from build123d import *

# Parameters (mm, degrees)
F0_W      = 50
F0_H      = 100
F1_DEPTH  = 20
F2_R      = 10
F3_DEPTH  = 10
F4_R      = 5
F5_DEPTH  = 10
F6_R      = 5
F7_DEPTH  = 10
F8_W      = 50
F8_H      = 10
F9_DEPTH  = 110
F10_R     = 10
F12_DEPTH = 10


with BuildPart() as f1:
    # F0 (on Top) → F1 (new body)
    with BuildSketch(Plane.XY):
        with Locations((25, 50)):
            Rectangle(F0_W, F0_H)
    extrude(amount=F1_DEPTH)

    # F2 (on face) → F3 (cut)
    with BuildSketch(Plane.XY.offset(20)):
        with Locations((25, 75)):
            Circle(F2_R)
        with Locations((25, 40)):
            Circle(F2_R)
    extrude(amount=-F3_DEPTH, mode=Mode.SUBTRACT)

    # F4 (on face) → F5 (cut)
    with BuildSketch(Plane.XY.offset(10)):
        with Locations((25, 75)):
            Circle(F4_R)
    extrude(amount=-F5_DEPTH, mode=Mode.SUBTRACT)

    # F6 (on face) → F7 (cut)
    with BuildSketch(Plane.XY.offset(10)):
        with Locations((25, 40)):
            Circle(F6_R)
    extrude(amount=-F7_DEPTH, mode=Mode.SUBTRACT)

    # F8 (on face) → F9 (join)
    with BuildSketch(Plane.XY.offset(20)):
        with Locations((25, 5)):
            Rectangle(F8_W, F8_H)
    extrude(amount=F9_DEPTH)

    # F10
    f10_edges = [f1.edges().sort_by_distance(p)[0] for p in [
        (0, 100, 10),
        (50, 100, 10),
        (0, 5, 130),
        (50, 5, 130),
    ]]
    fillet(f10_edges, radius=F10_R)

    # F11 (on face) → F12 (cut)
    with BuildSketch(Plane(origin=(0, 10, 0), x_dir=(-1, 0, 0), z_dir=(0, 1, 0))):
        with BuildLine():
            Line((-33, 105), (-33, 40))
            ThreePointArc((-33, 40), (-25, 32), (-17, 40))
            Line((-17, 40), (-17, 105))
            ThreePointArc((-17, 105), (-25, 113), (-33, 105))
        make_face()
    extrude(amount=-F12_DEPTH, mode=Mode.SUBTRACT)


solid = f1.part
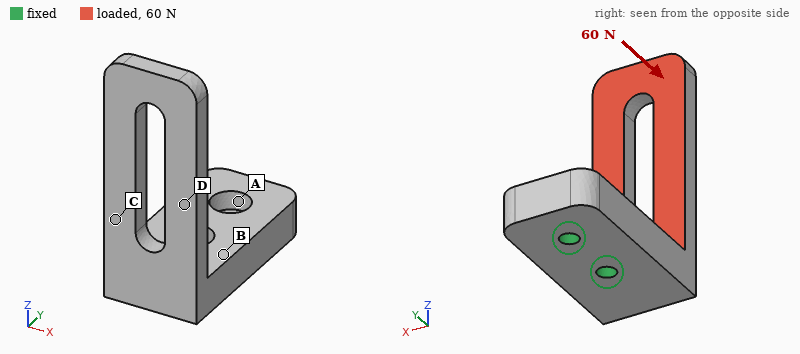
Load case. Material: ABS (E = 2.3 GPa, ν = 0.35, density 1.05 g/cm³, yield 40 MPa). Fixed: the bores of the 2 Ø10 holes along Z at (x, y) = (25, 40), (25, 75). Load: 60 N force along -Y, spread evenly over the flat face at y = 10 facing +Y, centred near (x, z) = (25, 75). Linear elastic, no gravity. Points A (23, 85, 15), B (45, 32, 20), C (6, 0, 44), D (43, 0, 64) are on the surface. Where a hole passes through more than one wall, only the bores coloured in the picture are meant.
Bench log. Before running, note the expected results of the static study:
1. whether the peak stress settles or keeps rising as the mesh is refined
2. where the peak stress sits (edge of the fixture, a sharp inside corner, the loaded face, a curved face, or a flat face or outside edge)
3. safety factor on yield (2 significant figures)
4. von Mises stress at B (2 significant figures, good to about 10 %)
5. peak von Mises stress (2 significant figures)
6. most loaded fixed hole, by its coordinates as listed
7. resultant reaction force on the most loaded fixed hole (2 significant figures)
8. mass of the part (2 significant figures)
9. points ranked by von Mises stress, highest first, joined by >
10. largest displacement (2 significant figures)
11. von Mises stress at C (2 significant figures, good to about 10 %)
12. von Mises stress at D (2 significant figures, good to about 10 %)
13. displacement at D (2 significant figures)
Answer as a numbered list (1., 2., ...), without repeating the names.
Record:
1. settles
2. the loaded face
3. 7.2
4. 1.4 MPa
5. 5.6 MPa
6. (25, 75)
7. 120 N
8. 140 g
9. C > D > B > A
10. 1.9 mm
11. 3.6 MPa
12. 2.2 MPa
13. 0.54 mm
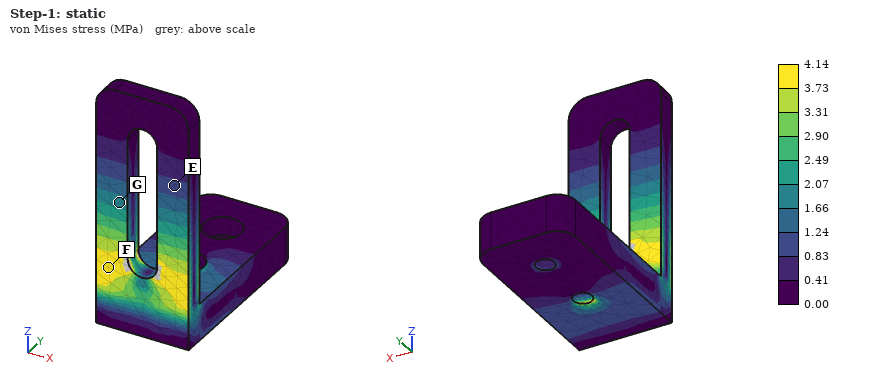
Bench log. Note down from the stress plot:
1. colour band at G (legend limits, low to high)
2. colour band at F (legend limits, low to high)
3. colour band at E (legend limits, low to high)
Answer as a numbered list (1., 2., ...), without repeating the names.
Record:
1. 1.66 to 2.07 MPa
2. 3.73 to 4.14 MPa
3. 0.83 to 1.24 MPa
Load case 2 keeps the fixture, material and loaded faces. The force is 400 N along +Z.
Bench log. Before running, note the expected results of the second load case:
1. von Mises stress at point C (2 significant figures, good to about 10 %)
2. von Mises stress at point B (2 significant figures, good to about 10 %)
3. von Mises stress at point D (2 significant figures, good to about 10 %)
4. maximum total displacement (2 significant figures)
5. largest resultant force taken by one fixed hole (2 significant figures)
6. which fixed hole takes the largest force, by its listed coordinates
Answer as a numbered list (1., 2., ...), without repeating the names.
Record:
1. 1.8 MPa
2. 3.0 MPa
3. 1.4 MPa
4. 0.67 mm
5. 640 N
6. (25, 40)
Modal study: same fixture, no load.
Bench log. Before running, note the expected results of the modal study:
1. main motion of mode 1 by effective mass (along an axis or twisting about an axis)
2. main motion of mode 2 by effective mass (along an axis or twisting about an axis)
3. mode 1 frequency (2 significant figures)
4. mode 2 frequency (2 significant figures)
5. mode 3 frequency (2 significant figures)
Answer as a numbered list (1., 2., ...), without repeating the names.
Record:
1. along Y
2. along X
3. 160 Hz
4. 300 Hz
5. 620 Hz
